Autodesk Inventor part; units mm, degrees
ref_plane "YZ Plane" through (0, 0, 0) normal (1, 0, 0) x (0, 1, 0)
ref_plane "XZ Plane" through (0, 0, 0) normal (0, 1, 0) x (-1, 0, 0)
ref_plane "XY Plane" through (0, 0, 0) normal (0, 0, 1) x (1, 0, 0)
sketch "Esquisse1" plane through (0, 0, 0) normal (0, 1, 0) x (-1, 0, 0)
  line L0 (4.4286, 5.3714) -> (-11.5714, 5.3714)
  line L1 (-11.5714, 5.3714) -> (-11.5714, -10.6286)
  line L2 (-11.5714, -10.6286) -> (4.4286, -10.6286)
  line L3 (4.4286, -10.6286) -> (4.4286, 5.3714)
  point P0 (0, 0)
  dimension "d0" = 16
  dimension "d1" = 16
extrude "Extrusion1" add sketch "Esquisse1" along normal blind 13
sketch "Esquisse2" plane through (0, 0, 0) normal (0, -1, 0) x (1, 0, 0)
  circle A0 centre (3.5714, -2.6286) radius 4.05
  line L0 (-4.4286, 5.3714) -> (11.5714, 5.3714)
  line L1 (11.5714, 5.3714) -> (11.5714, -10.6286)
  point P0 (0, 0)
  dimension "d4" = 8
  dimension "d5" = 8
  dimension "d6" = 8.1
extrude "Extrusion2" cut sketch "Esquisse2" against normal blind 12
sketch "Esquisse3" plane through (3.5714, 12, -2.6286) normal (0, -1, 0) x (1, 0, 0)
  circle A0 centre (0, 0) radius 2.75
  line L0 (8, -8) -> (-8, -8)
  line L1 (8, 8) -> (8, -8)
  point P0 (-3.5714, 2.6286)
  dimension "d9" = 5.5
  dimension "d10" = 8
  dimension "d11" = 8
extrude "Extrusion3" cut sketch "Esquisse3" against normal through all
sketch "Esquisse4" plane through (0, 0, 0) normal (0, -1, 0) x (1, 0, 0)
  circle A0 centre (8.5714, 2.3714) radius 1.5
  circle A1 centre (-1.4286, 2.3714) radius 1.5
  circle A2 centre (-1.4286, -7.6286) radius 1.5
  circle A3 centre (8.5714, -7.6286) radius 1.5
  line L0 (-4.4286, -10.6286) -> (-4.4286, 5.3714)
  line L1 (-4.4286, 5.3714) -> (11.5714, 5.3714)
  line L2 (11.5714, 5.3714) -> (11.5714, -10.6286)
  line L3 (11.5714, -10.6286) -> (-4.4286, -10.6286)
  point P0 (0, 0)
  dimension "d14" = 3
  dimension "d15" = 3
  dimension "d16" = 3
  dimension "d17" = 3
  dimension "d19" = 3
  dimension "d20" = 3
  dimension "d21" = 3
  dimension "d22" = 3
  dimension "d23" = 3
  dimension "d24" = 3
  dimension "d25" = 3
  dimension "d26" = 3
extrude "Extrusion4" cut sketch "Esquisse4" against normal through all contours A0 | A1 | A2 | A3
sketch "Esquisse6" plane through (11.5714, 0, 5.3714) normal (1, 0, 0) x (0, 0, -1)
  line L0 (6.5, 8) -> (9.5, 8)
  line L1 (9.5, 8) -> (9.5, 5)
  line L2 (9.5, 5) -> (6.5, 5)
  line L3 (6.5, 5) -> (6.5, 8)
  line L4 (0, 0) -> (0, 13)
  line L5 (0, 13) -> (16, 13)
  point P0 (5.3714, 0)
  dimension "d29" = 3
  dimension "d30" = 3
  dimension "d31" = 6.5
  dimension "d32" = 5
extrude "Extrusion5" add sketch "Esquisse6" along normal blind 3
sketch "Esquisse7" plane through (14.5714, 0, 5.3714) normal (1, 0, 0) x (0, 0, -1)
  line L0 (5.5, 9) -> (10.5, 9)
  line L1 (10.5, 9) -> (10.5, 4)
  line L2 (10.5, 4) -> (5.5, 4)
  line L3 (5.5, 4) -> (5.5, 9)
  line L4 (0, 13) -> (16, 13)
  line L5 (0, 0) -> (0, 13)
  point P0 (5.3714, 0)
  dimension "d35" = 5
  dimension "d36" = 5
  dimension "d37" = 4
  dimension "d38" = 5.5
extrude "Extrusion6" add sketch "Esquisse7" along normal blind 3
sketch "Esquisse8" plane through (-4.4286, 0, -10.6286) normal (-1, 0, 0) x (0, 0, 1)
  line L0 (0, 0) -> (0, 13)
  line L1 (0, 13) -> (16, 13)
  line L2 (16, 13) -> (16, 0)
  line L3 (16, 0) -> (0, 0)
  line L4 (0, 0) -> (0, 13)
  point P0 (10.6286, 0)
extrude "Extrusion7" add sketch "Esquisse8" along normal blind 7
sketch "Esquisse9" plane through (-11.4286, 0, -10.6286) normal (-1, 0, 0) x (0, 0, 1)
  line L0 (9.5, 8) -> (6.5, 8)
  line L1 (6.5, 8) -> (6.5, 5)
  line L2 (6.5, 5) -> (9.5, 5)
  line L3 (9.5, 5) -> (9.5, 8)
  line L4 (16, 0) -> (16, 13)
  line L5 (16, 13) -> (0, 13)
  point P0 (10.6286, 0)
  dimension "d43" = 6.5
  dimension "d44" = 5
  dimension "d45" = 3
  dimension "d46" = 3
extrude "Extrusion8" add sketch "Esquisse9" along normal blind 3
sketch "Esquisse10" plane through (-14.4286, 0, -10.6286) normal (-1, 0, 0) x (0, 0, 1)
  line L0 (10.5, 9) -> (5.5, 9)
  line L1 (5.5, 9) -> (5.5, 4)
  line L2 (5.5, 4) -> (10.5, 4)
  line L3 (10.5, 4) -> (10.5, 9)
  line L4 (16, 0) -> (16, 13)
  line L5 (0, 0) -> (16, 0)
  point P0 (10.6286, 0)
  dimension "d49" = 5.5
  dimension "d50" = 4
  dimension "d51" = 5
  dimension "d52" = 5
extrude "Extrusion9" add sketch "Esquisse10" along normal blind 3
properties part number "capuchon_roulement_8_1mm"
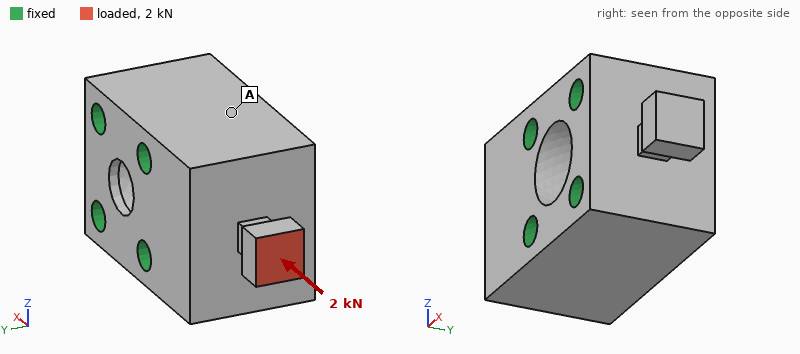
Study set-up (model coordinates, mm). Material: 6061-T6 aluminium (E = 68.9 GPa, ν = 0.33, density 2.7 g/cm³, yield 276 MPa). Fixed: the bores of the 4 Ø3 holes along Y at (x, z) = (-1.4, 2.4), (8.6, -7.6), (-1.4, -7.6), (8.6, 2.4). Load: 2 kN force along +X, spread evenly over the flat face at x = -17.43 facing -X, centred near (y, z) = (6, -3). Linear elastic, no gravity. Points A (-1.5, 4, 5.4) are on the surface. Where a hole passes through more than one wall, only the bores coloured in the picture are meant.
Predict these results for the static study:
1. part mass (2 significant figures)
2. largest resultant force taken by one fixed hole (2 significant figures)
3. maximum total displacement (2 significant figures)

11 g
1.1 kN
22 µm
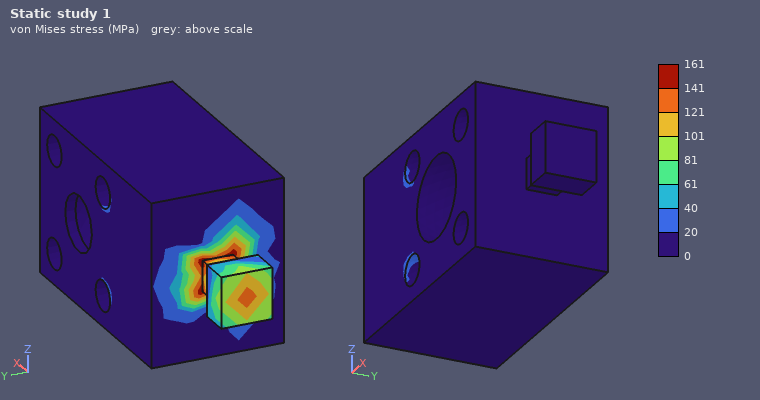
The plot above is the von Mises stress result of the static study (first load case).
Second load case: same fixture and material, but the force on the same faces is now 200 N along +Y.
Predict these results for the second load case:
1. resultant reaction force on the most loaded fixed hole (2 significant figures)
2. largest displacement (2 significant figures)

100 N
49 µm
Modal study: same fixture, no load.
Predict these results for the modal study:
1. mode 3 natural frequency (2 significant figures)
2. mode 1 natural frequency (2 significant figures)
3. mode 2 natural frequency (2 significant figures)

30 kHz
29 kHz
30 kHz
